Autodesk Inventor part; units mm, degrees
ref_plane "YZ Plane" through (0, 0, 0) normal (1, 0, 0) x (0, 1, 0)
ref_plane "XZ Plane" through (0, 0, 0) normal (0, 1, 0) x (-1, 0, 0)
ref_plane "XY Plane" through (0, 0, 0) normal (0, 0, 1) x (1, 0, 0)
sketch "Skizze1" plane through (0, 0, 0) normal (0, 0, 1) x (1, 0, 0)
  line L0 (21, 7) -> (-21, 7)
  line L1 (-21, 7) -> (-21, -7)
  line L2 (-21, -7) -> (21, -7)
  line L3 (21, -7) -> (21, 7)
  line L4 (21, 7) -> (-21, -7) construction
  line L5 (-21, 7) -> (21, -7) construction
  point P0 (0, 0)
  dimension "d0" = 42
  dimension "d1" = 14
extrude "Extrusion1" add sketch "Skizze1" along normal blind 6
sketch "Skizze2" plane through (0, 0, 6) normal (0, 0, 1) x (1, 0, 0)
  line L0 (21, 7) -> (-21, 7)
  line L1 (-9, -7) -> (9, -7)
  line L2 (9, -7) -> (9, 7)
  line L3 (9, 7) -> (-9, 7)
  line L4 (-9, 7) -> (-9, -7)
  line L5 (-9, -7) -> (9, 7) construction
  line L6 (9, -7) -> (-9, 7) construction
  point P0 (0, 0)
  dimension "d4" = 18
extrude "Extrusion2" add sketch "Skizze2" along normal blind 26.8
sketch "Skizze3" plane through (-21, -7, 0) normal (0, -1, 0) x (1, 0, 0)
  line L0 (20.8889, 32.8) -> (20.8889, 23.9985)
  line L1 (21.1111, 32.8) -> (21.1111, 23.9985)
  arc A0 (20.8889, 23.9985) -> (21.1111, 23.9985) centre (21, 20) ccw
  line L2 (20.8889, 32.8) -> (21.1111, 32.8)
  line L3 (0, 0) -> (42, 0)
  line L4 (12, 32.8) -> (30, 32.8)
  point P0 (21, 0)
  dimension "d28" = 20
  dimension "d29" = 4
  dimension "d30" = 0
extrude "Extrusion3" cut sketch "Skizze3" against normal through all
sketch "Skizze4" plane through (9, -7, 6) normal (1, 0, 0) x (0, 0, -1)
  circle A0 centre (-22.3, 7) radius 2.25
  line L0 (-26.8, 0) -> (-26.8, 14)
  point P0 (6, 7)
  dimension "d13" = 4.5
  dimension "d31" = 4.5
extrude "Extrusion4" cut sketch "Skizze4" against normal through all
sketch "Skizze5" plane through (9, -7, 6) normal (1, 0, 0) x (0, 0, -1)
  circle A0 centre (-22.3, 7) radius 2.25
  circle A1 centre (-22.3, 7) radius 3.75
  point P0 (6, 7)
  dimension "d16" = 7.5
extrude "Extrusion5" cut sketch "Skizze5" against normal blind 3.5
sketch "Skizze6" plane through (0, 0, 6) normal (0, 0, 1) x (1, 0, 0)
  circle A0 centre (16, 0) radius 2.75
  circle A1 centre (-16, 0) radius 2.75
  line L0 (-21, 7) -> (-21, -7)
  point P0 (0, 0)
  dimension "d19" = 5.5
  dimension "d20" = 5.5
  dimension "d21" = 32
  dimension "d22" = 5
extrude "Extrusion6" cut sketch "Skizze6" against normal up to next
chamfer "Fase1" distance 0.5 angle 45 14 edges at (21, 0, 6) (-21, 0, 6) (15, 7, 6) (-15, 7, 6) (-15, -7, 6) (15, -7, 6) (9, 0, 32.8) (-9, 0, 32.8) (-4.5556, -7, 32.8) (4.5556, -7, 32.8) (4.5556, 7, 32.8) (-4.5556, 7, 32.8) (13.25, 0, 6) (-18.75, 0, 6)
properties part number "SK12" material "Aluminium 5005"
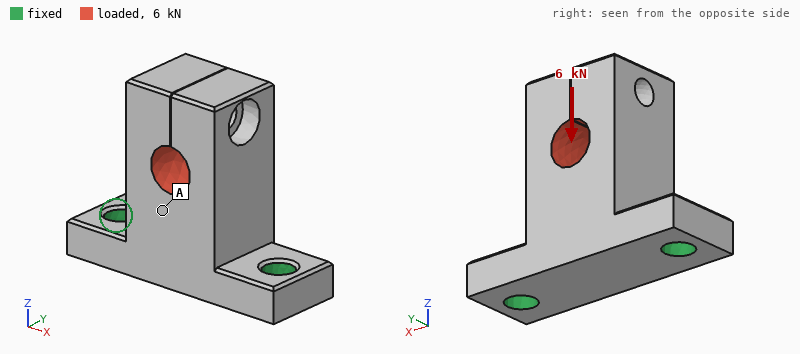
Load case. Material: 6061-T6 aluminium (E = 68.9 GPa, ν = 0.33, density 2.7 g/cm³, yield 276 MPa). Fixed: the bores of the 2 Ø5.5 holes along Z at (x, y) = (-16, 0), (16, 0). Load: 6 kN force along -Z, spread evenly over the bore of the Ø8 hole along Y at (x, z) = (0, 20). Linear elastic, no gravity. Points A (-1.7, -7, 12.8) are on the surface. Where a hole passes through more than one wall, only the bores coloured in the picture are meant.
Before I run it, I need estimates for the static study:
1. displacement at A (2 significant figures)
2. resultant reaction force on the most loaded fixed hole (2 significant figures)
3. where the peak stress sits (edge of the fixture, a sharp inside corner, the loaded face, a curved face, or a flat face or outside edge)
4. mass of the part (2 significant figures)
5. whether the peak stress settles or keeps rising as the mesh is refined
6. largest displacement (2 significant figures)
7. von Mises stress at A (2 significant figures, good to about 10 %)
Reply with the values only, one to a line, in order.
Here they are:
26 µm
3.3 kN
edge of the fixture
24 g
keeps rising
86 µm
32 MPa
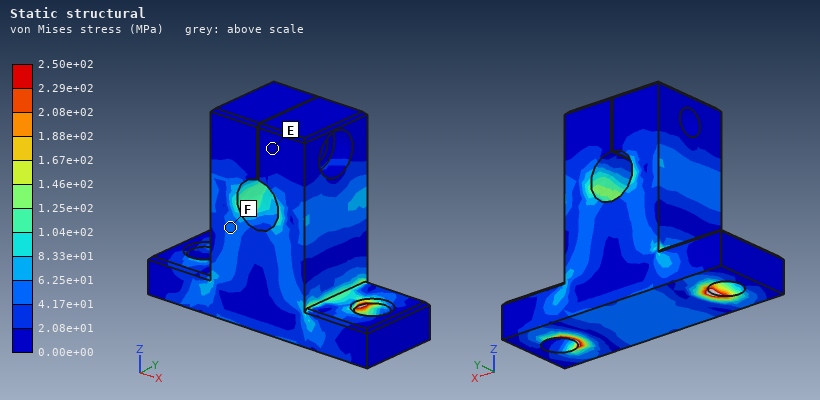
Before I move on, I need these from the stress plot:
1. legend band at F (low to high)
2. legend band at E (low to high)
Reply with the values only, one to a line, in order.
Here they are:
4.17e+01 to 6.25e+01 MPa
0.00e+00 to 2.08e+01 MPa
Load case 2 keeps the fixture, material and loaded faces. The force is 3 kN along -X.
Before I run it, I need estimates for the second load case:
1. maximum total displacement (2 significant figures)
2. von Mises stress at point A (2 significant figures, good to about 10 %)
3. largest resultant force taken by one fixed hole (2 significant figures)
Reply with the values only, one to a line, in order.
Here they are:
92 µm
50 MPa
2.6 kN
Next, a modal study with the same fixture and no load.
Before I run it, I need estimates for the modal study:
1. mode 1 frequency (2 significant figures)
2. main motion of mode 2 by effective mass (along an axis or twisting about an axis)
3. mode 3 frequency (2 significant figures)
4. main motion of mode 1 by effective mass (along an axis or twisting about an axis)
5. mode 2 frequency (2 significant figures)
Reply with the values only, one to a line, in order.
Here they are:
5100 Hz
along X
10 kHz
along Y
8300 Hz
